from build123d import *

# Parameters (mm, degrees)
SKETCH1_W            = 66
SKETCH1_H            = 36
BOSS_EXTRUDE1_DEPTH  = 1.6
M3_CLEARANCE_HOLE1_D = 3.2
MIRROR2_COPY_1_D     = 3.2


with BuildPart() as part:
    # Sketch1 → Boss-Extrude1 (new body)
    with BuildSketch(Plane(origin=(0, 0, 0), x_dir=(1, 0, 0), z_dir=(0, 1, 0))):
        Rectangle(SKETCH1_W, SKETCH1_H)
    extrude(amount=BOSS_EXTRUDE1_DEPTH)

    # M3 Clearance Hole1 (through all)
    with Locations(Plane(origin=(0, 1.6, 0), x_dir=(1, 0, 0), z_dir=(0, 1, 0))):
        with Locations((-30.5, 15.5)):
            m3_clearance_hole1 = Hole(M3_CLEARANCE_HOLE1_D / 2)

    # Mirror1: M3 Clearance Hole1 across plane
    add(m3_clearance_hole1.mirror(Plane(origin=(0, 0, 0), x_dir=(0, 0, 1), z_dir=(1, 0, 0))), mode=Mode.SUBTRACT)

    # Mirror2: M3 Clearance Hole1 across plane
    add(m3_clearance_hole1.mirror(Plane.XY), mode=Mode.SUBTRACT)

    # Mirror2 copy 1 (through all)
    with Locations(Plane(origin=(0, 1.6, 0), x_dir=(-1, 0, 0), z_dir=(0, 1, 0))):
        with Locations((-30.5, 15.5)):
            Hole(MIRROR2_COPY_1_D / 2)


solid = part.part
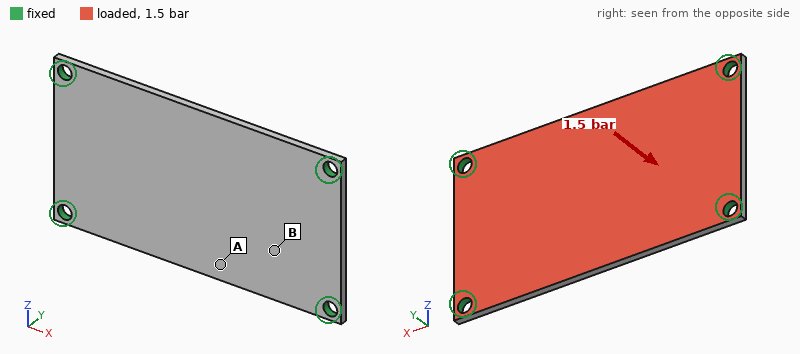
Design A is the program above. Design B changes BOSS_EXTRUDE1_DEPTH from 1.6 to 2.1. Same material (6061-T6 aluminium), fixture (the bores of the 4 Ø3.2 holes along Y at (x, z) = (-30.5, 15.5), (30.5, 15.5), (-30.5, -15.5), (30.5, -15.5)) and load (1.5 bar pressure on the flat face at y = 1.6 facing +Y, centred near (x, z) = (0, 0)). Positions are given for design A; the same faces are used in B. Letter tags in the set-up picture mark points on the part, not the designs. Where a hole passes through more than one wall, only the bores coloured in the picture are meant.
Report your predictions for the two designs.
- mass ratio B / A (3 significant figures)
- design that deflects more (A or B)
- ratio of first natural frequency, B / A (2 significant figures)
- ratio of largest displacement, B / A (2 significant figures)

1.31
A
1.3
0.46
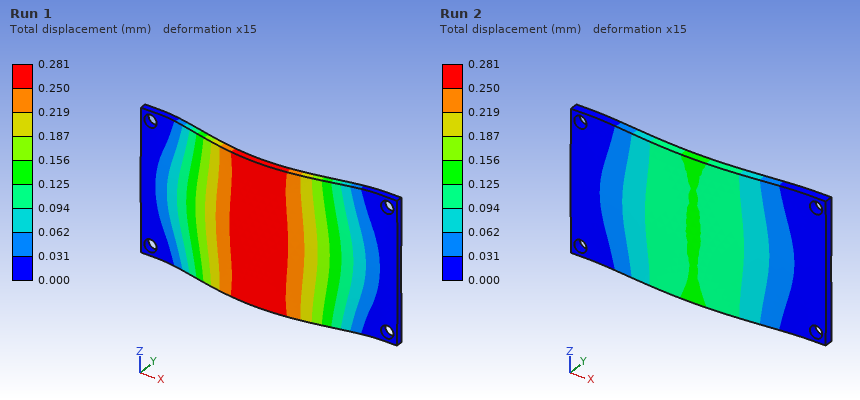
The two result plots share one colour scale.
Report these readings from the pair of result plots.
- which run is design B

Run 2
